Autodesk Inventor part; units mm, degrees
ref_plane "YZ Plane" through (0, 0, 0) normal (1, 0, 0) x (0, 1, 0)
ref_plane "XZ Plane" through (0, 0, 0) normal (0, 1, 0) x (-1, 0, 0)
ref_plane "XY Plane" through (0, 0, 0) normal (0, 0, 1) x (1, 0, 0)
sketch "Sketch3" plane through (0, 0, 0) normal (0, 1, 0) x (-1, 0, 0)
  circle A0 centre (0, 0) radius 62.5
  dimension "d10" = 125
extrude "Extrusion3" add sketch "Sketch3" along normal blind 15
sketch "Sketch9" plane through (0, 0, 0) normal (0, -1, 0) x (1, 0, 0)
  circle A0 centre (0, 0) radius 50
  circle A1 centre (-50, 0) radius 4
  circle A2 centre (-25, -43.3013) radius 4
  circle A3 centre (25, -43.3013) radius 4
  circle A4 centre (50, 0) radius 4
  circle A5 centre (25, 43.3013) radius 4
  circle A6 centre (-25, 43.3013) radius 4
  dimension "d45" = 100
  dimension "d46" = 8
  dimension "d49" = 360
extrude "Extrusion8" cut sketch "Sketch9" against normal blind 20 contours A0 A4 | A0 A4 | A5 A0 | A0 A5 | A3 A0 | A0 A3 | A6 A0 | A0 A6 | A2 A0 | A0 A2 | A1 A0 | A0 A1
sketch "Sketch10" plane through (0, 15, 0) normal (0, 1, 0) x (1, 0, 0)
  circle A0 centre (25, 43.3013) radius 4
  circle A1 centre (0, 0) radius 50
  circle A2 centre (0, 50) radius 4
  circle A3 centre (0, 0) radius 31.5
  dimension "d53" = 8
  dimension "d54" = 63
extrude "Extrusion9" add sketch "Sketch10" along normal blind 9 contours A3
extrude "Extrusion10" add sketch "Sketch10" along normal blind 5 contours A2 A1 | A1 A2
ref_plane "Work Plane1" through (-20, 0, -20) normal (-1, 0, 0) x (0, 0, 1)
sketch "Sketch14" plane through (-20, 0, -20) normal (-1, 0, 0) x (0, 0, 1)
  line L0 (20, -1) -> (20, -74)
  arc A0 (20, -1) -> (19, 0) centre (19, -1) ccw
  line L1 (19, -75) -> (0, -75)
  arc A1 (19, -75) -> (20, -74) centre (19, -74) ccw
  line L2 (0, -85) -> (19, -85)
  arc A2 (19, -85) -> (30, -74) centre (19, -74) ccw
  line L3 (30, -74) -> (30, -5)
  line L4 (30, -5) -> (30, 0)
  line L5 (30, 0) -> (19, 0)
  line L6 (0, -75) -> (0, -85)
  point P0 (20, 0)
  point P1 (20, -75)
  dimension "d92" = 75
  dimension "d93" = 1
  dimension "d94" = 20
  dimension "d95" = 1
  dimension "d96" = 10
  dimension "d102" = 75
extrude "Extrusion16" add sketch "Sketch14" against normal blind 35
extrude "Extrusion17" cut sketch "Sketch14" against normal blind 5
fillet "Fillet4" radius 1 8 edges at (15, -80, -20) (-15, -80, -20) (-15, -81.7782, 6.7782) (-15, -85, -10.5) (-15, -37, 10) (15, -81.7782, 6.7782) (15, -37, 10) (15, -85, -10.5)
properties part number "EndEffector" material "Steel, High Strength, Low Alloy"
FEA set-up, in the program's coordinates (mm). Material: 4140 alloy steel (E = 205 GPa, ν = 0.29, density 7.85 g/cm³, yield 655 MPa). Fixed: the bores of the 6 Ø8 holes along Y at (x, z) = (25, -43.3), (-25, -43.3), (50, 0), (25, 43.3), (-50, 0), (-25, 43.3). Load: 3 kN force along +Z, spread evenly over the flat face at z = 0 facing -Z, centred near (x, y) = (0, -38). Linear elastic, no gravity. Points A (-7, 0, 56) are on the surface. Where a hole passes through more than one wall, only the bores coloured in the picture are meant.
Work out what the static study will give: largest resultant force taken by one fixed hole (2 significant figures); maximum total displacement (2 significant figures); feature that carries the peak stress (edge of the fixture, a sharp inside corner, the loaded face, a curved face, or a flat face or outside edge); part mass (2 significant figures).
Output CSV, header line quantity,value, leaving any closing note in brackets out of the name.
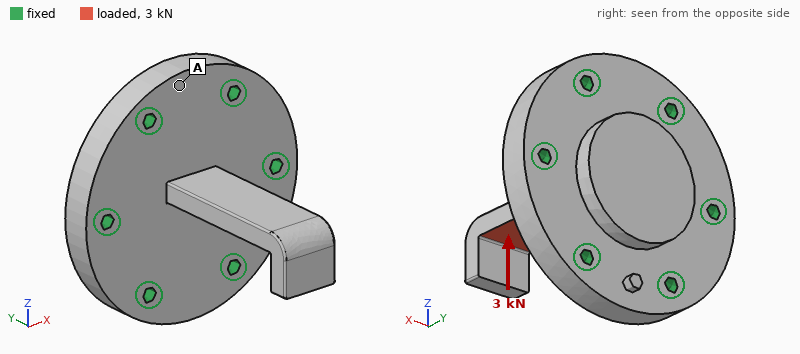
quantity,value
largest resultant force taken by one fixed hole,1.3 kN
maximum total displacement,0.45 mm
feature that carries the peak stress,the loaded face
part mass,1.9 kg
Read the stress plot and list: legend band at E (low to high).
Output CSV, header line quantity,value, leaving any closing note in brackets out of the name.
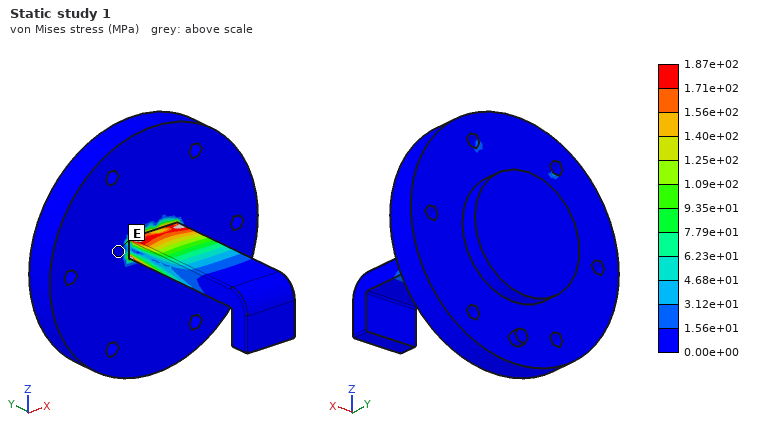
quantity,value
legend band at E,0.00e+00 to 1.56e+01 MPa
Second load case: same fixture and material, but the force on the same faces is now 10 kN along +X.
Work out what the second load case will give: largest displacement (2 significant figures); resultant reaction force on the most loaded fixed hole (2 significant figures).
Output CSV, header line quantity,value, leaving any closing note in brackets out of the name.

quantity,value
largest displacement,0.29 mm
resultant reaction force on the most loaded fixed hole,4.3 kN
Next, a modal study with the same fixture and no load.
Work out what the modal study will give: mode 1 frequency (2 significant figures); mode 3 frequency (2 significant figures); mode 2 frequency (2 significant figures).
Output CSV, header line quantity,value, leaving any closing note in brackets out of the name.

quantity,value
mode 1 frequency,810 Hz
mode 3 frequency,3800 Hz
mode 2 frequency,2000 Hz
